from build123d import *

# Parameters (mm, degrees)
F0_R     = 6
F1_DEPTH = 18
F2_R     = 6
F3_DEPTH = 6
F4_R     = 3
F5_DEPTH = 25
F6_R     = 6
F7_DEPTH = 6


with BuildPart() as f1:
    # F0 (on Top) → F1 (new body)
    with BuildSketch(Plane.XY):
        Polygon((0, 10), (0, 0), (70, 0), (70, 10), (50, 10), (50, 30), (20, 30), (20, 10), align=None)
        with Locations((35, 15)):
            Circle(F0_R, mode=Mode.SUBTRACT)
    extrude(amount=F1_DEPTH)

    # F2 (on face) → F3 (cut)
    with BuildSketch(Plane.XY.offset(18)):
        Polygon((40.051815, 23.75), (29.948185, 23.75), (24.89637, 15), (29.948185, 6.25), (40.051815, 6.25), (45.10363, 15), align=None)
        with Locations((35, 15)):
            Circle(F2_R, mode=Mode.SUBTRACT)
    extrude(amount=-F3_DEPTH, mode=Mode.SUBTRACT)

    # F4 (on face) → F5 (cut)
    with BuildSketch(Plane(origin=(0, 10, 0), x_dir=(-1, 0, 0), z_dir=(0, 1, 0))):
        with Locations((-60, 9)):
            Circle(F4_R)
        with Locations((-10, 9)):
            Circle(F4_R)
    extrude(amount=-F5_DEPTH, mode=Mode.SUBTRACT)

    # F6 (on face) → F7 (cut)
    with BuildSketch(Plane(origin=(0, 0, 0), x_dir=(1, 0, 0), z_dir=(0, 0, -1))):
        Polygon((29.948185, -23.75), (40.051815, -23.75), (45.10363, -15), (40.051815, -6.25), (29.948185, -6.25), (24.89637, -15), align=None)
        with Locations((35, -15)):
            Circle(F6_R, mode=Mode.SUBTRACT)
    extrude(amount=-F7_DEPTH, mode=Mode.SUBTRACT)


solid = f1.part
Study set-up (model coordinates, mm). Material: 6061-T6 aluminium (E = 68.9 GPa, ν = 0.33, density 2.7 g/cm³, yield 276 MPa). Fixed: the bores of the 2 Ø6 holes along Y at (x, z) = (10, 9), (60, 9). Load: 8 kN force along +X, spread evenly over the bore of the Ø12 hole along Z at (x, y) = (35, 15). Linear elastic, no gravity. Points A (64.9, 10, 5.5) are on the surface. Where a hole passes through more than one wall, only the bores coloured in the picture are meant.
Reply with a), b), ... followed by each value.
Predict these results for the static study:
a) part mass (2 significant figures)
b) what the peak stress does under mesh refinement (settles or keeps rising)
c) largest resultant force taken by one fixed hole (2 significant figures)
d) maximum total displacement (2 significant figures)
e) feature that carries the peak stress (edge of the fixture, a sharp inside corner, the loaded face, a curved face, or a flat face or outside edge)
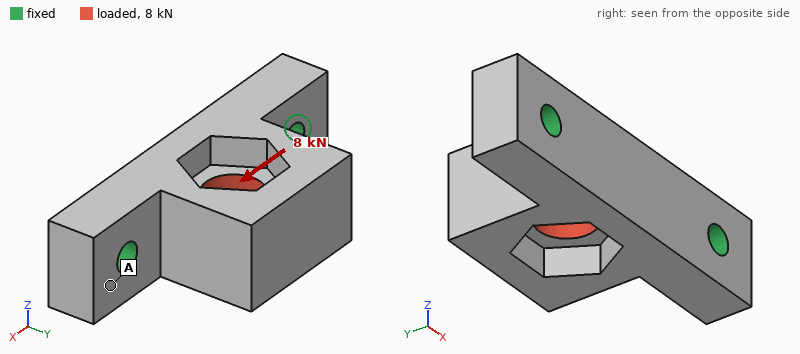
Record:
a) 51 g
b) keeps rising
c) 4.4 kN
d) 32 µm
e) edge of the fixture
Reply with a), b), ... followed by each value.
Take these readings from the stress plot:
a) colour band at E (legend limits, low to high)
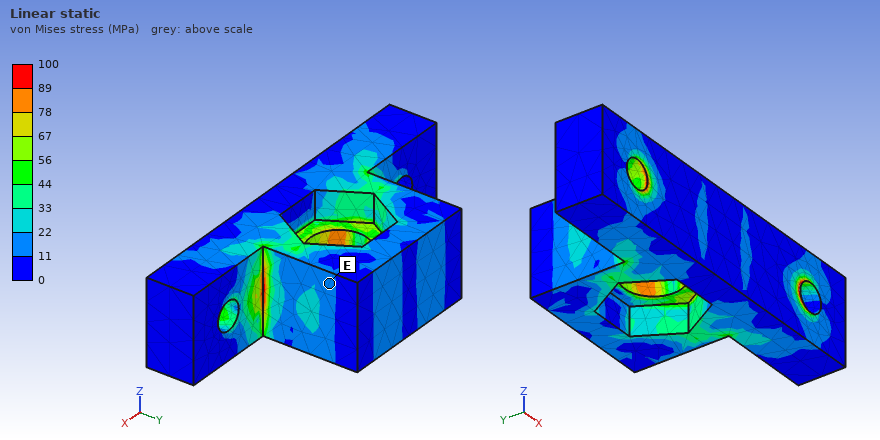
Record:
a) 11 to 22 MPa
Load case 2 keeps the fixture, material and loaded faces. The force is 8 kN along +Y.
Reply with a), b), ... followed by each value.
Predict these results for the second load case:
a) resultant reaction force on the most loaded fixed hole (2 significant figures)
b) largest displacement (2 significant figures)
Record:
a) 4.0 kN
b) 37 µm
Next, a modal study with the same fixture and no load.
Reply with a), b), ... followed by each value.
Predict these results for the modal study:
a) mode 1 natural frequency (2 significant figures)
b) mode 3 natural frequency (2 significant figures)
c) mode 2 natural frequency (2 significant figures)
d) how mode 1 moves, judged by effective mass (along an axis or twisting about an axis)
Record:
a) 7000 Hz
b) 15 kHz
c) 14 kHz
d) along Z
